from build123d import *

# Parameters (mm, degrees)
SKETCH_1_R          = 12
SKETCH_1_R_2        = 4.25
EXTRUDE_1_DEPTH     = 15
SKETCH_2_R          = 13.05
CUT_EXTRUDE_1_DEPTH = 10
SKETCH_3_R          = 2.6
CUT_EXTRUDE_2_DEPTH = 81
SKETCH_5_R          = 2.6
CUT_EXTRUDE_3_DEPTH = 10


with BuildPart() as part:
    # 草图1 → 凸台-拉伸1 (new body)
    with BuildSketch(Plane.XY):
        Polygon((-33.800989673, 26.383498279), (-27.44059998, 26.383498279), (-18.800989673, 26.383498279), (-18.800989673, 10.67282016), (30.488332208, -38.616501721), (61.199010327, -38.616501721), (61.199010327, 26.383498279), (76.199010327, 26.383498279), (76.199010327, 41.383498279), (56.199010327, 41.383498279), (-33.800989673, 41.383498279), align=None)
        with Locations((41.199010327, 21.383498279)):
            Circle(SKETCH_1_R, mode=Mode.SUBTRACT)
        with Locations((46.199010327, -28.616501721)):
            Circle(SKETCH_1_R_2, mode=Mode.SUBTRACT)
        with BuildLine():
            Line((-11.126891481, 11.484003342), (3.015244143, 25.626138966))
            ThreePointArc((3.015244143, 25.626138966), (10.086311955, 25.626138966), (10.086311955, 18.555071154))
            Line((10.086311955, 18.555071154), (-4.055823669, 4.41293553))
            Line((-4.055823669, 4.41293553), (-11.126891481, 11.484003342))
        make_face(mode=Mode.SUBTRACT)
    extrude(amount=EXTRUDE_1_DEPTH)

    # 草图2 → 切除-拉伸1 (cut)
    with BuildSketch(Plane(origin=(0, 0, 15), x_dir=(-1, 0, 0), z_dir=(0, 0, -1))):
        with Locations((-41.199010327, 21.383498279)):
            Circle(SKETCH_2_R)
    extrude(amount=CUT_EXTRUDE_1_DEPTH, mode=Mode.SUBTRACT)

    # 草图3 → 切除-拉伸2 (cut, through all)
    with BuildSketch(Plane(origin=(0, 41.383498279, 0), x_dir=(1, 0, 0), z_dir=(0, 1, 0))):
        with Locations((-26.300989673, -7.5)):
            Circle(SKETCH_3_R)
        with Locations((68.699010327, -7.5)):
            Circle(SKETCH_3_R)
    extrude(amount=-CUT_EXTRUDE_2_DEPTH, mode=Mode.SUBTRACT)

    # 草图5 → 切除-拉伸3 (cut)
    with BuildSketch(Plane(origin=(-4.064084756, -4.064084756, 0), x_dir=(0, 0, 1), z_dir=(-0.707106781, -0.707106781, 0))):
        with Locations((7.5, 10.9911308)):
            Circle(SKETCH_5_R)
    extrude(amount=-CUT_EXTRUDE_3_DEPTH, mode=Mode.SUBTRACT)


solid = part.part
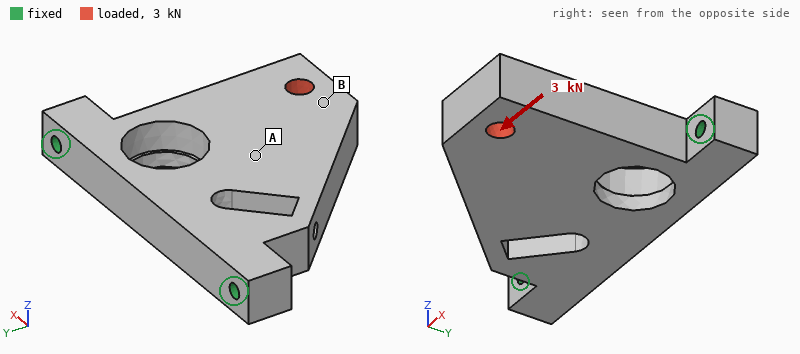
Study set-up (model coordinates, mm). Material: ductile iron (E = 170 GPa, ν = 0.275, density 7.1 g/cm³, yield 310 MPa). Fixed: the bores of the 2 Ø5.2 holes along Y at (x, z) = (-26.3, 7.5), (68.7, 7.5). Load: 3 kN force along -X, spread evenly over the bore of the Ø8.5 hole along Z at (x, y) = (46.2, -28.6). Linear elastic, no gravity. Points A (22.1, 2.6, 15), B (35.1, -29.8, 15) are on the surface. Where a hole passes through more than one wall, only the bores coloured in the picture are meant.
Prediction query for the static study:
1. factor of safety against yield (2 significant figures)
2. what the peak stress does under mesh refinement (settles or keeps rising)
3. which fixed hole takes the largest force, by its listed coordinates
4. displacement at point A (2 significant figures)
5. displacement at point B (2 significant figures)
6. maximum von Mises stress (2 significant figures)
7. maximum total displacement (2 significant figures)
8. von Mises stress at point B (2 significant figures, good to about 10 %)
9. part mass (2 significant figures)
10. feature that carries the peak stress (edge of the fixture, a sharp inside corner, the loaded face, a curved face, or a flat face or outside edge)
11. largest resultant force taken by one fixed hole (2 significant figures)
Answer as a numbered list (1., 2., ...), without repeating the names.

1. 3.4
2. settles
3. (-26.3, 7.5)
4. 7.2 µm
5. 14 µm
6. 91 MPa
7. 18 µm
8. 9.9 MPa
9. 510 g
10. a curved face
11. 3.0 kN
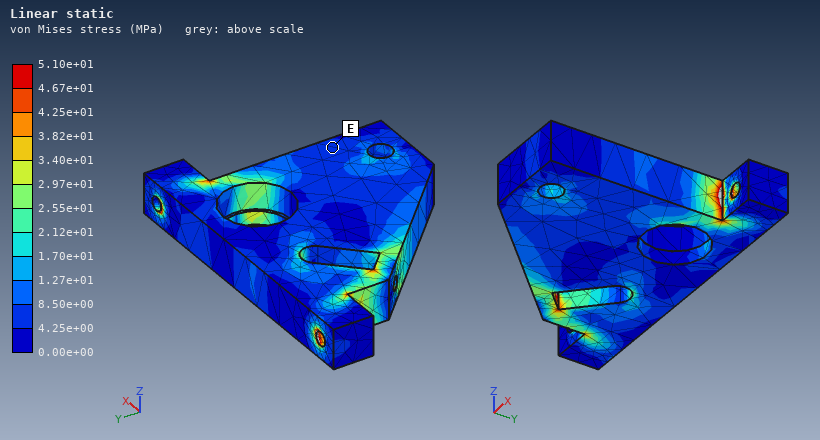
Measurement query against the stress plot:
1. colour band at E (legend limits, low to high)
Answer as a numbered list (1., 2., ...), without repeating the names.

1. 4.25e+00 to 8.50e+00 MPa
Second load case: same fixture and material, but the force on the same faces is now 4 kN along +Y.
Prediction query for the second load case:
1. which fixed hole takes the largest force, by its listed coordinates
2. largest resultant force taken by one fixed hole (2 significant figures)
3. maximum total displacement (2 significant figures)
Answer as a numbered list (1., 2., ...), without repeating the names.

1. (68.7, 7.5)
2. 3.2 kN
3. 10 µm
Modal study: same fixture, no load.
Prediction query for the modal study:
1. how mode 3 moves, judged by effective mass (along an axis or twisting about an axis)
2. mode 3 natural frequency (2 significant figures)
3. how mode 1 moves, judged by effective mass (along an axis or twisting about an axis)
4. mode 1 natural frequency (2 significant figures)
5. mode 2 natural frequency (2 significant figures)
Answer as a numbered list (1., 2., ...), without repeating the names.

1. along X
2. 5500 Hz
3. along Z
4. 1300 Hz
5. 4800 Hz
